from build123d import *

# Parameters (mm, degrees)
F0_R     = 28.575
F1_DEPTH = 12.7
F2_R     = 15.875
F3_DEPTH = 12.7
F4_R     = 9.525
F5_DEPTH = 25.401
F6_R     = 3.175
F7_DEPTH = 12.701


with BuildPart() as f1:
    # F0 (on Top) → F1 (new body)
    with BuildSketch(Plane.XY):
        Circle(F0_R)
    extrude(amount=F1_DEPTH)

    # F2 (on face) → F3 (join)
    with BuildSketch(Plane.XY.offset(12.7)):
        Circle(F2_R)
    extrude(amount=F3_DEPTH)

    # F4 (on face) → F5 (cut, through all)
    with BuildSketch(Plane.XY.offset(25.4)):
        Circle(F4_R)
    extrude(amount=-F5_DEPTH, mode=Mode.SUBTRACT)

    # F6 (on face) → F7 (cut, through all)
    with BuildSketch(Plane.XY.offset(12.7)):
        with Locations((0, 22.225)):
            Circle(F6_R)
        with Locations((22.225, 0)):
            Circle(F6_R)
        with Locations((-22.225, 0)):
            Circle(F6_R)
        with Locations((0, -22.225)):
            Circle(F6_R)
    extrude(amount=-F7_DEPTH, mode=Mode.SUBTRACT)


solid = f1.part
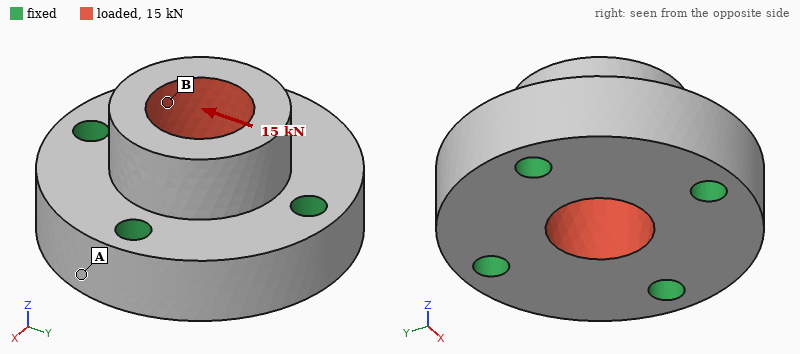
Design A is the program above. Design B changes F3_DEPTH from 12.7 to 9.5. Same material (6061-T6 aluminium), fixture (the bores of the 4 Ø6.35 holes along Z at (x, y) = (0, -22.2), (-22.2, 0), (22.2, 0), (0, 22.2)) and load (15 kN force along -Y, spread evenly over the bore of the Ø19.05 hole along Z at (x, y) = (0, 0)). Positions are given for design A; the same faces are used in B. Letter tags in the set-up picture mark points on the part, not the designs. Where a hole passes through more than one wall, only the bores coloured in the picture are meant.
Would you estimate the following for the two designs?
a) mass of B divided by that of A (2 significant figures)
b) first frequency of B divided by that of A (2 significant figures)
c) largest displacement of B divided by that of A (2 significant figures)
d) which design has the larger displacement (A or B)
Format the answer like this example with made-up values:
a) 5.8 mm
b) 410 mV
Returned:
a) 0.95
b) 1.1
c) 0.76
d) A
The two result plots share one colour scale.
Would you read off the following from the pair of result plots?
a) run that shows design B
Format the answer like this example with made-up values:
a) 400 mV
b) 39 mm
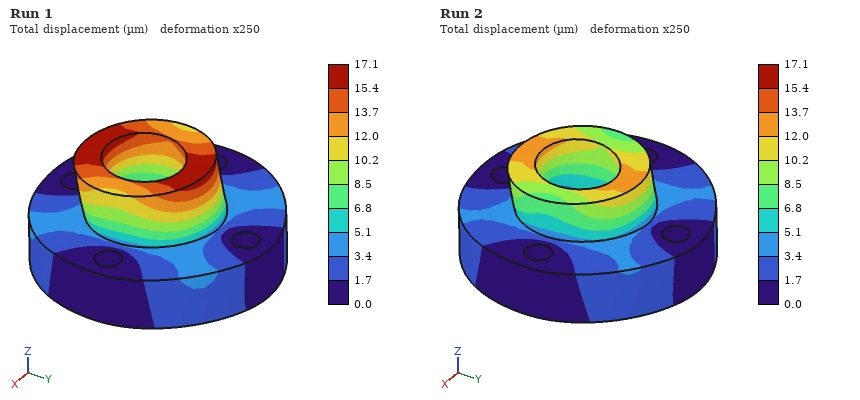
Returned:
a) Run 2
